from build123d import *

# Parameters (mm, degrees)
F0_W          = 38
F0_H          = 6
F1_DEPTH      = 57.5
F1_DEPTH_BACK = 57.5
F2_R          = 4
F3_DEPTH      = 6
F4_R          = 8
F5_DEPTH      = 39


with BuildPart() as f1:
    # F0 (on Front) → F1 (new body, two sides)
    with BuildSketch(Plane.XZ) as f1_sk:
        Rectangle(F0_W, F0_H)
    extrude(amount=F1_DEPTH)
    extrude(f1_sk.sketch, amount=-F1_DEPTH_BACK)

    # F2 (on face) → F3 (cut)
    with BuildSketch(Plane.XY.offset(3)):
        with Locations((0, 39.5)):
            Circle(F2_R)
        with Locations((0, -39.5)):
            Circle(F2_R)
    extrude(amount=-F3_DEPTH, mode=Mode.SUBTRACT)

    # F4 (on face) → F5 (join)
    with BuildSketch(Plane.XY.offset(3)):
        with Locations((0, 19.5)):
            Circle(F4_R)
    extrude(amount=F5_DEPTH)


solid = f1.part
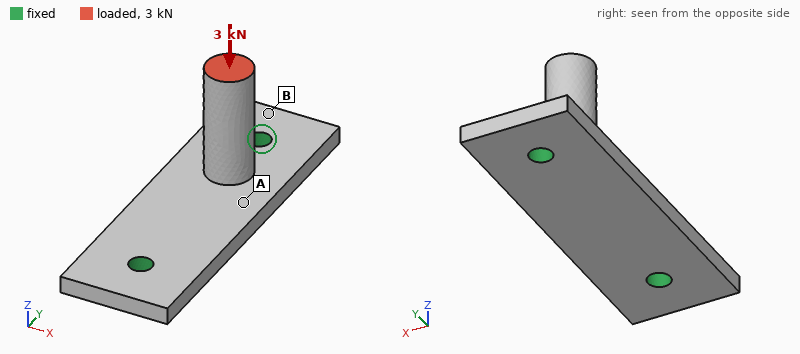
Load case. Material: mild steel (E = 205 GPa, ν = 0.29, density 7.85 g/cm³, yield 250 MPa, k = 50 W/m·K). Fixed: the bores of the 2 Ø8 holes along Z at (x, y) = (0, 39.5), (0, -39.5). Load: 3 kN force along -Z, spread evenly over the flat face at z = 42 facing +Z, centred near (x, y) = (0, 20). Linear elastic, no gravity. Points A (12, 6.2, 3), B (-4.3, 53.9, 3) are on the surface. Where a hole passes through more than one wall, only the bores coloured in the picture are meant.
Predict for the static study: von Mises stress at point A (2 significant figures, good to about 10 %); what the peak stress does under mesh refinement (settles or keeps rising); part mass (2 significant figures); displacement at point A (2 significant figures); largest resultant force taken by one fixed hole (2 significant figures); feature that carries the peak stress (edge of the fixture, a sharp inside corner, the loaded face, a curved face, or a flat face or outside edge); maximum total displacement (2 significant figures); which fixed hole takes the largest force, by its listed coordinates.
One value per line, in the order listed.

47 MPa
keeps rising
260 g
29 µm
2.5 kN
edge of the fixture
57 µm
(0, 39.5)
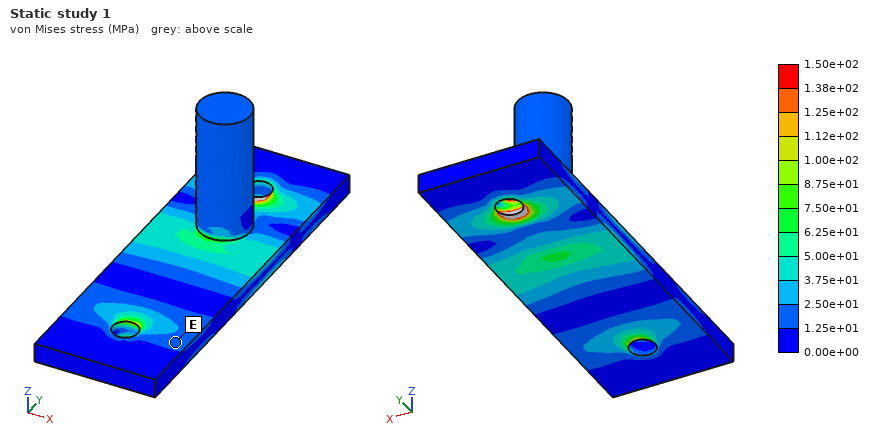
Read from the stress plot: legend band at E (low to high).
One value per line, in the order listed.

1.25e+01 to 2.50e+01 MPa
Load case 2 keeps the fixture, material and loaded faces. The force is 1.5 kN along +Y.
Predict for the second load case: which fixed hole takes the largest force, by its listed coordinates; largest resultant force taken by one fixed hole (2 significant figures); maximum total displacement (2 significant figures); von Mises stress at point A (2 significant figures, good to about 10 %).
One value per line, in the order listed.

(0, 39.5)
1.4 kN
0.16 mm
85 MPa
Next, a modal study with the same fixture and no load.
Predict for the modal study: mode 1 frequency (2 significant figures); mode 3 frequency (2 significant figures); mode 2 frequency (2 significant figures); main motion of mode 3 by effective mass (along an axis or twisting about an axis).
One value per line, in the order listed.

2900 Hz
6700 Hz
3000 Hz
along Z
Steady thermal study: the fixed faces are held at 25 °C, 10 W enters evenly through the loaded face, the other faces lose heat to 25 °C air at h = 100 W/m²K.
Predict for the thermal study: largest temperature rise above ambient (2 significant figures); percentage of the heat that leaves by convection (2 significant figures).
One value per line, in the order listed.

37 K
60 %
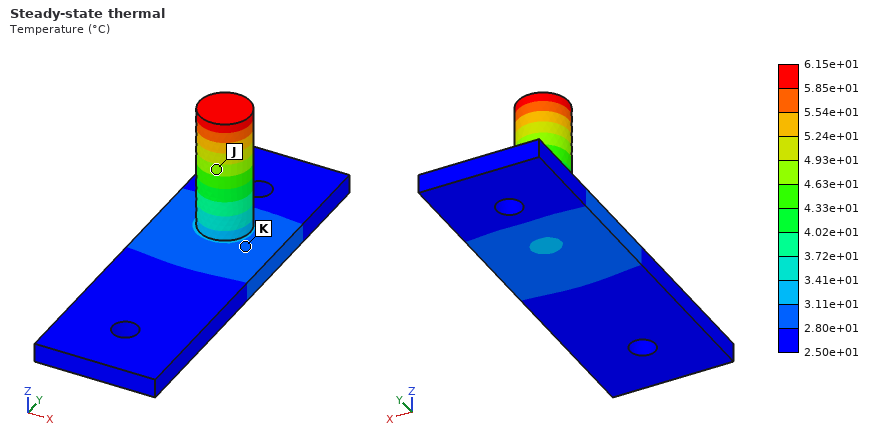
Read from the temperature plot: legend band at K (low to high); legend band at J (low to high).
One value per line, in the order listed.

2.80e+01 to 3.11e+01 °C
4.63e+01 to 4.93e+01 °C
